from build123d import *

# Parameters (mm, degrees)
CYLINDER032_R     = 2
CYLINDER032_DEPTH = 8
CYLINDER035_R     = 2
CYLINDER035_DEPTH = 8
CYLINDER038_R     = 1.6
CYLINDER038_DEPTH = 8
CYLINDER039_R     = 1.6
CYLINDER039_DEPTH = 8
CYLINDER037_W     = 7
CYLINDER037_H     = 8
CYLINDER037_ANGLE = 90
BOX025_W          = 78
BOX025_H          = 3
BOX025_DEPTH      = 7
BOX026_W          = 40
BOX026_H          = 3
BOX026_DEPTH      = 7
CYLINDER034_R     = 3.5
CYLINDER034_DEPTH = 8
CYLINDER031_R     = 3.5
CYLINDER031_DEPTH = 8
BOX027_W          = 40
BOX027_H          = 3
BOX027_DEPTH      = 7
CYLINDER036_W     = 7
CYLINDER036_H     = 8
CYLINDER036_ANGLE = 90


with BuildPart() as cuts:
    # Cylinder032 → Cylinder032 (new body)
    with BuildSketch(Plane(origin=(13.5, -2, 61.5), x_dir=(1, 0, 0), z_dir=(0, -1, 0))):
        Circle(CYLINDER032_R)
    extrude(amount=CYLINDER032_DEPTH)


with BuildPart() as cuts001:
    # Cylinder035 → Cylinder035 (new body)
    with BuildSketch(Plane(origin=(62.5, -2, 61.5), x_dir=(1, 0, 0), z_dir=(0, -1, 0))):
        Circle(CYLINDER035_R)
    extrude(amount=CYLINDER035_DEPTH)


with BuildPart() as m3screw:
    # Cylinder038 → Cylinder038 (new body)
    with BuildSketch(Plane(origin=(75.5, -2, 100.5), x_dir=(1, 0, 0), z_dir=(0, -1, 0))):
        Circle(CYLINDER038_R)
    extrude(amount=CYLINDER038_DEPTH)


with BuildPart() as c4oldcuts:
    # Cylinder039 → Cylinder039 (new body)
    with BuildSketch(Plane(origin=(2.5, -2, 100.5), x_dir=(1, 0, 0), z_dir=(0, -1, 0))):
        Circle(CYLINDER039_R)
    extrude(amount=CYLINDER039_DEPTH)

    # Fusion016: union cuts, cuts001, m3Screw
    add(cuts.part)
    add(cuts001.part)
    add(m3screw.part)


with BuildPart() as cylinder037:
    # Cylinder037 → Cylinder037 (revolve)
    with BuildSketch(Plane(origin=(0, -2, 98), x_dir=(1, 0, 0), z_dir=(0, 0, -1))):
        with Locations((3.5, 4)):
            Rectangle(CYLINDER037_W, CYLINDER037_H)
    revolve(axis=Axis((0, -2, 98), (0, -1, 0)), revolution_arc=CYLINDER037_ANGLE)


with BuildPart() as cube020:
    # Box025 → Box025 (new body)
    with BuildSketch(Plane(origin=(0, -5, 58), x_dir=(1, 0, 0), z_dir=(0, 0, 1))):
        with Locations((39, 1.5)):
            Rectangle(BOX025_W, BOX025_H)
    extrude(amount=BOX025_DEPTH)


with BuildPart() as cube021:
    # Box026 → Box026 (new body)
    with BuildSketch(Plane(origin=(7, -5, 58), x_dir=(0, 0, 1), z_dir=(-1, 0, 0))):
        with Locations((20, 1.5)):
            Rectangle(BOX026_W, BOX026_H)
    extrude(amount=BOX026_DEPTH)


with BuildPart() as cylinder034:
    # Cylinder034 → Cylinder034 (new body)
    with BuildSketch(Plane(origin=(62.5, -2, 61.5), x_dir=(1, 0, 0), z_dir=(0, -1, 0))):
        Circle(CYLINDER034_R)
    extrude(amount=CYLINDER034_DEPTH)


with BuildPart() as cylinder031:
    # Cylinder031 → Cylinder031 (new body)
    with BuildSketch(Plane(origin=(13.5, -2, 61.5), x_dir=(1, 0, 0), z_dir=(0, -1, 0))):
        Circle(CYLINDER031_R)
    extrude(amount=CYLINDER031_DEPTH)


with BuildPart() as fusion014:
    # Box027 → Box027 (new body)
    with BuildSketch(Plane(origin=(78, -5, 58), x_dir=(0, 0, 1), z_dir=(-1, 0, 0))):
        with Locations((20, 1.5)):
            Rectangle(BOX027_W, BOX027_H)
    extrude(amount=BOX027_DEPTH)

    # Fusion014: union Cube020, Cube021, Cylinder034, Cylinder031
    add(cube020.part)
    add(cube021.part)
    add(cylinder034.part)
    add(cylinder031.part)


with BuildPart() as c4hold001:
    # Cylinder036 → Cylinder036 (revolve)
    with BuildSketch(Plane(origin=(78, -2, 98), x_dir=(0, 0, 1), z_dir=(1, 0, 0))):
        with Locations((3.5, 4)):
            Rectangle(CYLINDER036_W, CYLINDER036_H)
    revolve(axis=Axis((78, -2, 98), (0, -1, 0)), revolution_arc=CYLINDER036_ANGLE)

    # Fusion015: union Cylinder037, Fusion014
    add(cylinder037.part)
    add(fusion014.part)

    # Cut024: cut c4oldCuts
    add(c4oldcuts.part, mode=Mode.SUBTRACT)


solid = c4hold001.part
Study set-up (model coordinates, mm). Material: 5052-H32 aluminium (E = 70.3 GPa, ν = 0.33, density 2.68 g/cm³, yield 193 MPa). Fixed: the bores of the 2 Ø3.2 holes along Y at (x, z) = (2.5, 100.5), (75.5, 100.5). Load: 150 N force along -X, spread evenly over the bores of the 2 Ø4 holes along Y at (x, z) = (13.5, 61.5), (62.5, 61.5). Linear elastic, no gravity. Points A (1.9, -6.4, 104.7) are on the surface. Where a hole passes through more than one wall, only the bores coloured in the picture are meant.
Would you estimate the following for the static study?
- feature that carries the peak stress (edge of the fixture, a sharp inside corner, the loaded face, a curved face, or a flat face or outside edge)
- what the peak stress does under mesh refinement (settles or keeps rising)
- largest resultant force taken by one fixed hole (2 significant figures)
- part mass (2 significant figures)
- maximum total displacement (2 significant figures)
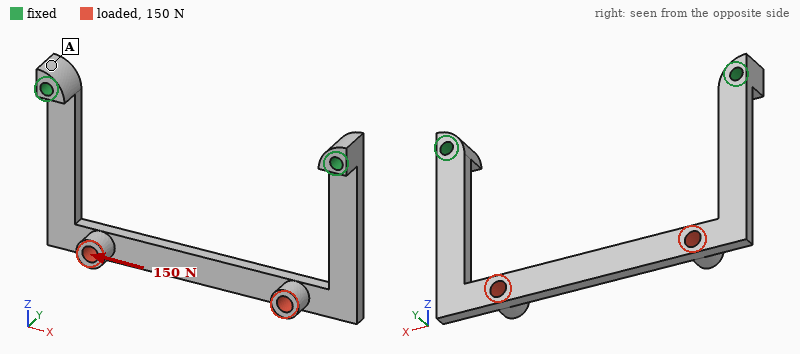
edge of the fixture
keeps rising
82 N
9.9 g
0.12 mm
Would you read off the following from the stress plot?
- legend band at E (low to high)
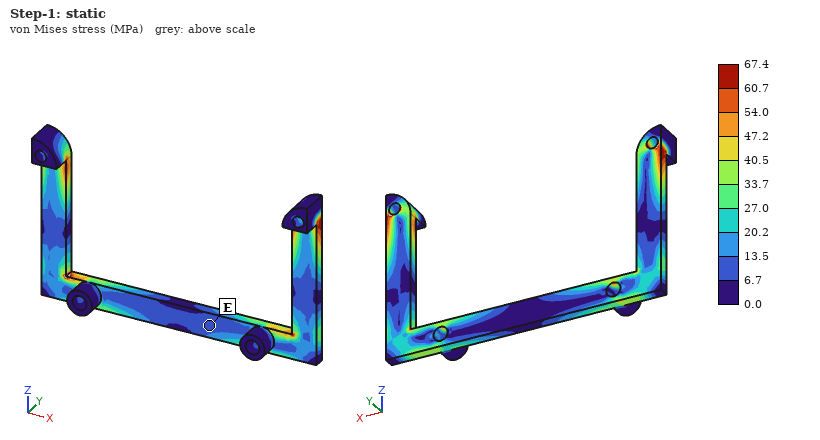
6.7 to 13.5 MPa
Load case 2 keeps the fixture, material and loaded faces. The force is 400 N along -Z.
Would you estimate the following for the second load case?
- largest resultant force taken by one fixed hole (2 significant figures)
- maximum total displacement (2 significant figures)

210 N
0.42 mm
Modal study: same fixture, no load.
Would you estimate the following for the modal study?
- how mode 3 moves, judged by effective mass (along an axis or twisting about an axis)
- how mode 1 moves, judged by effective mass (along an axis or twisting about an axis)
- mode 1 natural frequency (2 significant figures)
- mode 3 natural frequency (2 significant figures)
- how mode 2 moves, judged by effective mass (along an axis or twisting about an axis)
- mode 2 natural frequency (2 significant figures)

along X
along Y
710 Hz
2400 Hz
twisting about Z
1500 Hz
